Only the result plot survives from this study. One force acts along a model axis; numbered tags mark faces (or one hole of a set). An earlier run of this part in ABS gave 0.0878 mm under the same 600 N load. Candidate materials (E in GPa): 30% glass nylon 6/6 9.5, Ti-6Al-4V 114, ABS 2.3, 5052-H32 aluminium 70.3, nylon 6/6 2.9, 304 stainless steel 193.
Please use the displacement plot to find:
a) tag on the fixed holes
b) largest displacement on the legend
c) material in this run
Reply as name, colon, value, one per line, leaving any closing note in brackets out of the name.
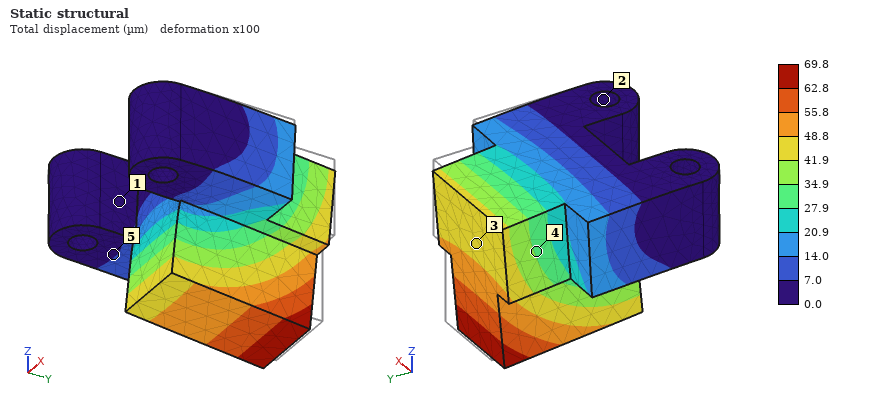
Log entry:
tag on the fixed holes: 2
largest displacement on the legend: 69.8 µm
material in this run: nylon 6/6
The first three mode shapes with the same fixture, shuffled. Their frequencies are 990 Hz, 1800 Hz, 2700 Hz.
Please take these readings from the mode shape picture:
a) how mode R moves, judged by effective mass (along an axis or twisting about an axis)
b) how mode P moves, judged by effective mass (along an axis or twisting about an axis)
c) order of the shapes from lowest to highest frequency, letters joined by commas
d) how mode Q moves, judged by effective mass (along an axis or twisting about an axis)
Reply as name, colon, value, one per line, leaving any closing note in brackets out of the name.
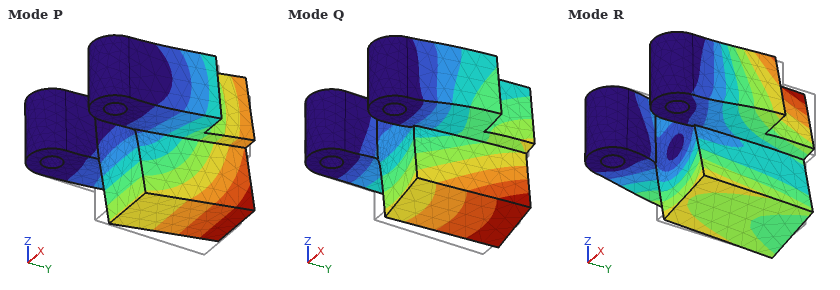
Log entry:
how mode R moves, judged by effective mass: along X
how mode P moves, judged by effective mass: along Z
order of the shapes from lowest to highest frequency, letters joined by commas: P, Q, R
how mode Q moves, judged by effective mass: along X
